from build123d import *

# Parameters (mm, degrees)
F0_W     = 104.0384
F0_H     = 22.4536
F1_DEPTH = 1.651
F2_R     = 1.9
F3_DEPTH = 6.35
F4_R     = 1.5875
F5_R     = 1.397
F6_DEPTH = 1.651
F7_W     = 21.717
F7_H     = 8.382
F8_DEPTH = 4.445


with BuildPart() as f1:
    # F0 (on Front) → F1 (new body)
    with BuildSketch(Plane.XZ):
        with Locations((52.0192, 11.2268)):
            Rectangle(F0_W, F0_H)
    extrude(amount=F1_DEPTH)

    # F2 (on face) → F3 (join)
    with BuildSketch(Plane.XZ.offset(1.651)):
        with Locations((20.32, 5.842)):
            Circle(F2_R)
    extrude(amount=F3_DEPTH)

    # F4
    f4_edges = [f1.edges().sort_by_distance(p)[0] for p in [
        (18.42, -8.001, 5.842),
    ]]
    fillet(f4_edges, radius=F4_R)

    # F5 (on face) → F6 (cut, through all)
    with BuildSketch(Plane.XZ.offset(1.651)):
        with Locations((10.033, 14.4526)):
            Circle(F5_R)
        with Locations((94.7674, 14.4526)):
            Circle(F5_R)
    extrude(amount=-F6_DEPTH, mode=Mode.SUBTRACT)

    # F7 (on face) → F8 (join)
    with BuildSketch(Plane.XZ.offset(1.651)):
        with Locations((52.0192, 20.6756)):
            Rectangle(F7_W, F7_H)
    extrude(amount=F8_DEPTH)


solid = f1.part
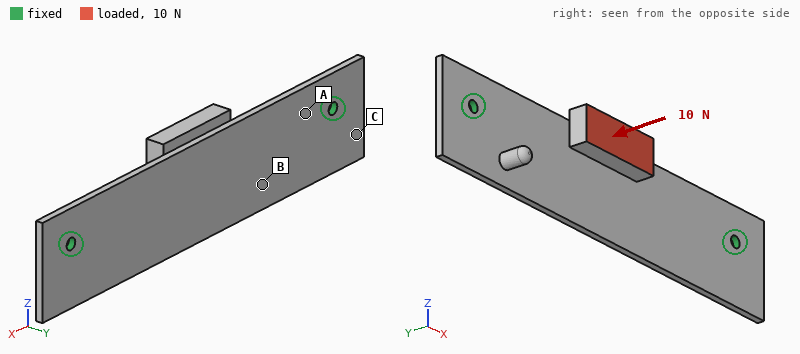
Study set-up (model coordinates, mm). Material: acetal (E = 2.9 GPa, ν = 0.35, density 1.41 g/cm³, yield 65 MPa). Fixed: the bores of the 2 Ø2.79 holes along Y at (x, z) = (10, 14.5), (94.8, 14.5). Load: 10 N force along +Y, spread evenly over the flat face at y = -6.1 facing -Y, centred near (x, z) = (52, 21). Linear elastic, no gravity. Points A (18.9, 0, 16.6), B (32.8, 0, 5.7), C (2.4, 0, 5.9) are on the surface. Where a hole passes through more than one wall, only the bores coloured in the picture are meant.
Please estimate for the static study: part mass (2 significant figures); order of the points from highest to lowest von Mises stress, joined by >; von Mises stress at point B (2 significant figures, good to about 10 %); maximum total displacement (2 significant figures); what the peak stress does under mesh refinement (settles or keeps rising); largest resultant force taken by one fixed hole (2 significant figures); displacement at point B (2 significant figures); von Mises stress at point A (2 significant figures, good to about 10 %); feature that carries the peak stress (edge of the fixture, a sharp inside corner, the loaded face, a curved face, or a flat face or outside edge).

6.6 g
A > B > C
3.1 MPa
1.1 mm
keeps rising
7.2 N
0.36 mm
5.4 MPa
edge of the fixture
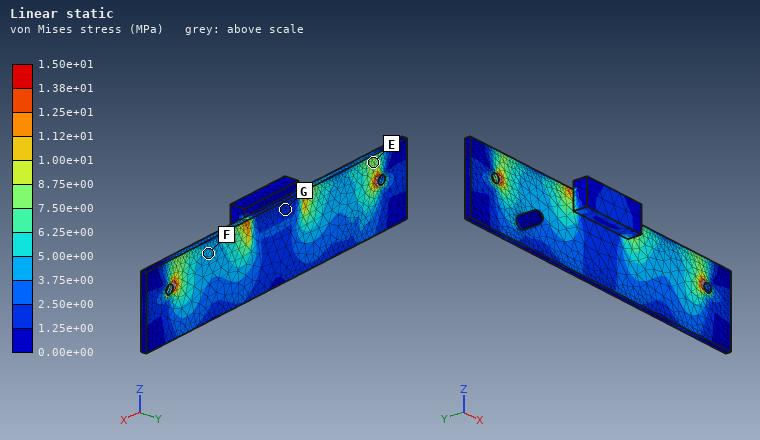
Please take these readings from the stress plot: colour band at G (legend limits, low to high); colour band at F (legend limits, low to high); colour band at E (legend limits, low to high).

1.25e+00 to 2.50e+00 MPa
3.75e+00 to 5.00e+00 MPa
7.50e+00 to 8.75e+00 MPa
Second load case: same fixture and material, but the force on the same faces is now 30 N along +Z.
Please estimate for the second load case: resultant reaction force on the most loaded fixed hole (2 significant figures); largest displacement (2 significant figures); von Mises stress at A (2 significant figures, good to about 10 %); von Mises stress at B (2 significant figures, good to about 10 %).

19 N
1.0 mm
6.7 MPa
4.3 MPa
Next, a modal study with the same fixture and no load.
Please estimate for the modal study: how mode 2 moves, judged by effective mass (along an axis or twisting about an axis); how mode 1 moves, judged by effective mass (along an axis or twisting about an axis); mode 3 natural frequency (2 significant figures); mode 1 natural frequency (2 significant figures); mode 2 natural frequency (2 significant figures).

twisting about X
along Y
850 Hz
310 Hz
550 Hz
